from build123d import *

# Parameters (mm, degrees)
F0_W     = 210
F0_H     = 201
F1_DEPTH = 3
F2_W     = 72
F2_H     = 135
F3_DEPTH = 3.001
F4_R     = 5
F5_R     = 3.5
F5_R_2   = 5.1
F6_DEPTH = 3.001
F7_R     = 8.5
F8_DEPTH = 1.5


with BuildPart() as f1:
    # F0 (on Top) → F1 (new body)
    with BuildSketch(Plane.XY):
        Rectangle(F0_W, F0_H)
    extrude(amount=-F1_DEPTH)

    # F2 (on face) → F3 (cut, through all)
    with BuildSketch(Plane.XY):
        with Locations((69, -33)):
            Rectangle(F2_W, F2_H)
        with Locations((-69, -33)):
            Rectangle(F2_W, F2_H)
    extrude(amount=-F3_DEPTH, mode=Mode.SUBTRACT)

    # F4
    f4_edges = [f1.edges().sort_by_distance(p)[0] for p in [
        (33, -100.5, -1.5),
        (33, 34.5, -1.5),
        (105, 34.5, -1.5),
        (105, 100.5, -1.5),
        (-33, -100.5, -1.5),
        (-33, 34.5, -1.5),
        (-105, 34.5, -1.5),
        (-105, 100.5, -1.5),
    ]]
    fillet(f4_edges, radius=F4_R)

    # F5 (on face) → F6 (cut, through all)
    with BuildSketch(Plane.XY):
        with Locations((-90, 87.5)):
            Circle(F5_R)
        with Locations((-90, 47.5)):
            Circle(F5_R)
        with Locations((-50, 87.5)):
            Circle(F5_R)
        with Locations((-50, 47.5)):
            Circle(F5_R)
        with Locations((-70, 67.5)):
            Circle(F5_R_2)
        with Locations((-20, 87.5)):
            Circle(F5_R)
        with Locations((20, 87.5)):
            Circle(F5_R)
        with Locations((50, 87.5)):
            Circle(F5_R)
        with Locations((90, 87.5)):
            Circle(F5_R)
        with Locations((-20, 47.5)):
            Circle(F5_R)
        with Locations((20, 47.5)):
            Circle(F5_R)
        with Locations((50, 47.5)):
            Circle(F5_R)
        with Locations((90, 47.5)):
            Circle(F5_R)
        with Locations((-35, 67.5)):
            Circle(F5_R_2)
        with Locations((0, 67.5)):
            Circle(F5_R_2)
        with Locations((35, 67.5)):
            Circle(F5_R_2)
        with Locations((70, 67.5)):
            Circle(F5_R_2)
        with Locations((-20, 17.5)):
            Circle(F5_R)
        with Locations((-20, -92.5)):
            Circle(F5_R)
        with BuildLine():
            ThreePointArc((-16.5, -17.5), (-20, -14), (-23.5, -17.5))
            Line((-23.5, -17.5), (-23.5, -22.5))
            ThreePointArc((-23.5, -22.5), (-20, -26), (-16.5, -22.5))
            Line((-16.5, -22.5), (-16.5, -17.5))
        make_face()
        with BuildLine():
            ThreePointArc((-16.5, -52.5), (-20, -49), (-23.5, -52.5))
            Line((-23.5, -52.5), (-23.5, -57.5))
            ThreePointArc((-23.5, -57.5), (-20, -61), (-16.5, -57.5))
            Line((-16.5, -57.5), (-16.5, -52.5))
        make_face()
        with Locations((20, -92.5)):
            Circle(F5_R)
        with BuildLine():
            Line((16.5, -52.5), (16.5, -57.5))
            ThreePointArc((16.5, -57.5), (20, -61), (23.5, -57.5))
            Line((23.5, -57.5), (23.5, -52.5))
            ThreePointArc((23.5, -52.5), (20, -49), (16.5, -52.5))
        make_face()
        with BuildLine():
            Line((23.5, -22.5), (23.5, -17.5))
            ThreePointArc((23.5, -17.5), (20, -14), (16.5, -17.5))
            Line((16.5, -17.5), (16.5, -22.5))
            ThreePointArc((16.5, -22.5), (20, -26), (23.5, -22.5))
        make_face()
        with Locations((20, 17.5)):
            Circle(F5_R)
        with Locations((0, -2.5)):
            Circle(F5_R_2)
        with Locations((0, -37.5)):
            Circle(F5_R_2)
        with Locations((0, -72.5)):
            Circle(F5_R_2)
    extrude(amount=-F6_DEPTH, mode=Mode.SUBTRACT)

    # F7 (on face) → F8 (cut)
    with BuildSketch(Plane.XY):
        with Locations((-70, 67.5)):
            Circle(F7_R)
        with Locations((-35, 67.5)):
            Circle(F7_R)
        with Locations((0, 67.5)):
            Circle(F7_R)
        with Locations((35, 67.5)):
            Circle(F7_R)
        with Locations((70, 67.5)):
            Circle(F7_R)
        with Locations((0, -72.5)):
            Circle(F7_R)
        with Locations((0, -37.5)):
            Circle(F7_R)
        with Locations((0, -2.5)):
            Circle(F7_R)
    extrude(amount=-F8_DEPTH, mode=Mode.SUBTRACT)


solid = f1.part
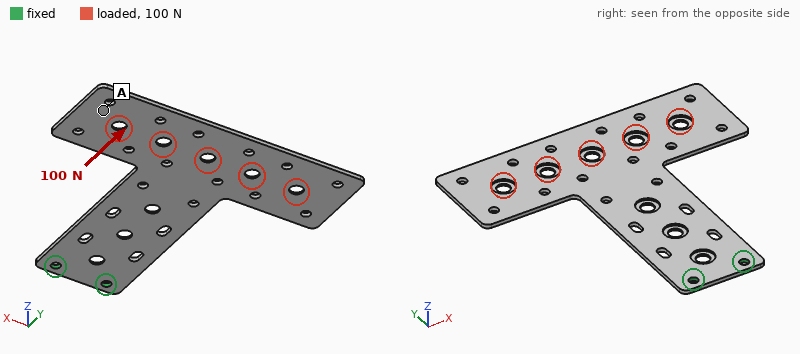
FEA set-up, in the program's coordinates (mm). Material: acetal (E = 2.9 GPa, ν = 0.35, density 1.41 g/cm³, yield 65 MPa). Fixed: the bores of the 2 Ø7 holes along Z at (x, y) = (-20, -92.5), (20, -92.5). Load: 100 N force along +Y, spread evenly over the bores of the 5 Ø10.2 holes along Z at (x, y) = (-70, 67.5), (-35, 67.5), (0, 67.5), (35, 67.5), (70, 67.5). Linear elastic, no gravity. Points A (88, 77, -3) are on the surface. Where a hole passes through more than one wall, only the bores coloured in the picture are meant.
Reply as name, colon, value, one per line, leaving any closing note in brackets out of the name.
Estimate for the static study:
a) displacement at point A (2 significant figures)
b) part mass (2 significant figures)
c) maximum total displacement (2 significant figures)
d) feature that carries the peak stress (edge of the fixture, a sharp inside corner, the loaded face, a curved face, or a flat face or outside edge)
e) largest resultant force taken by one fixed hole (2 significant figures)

displacement at point A: 2.7 mm
part mass: 87 g
maximum total displacement: 3.4 mm
feature that carries the peak stress: a curved face
largest resultant force taken by one fixed hole: 50 N
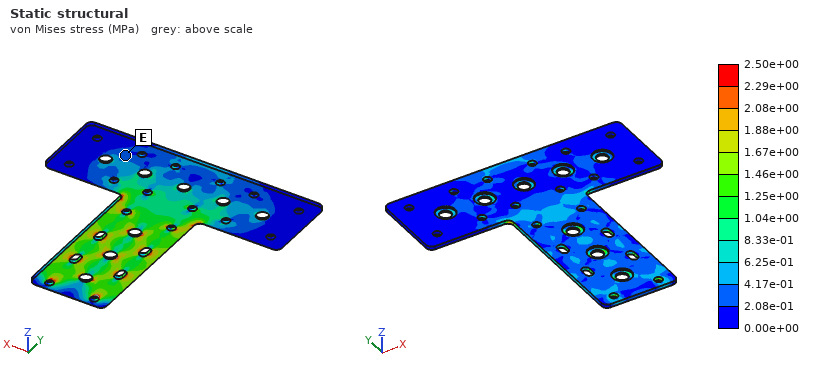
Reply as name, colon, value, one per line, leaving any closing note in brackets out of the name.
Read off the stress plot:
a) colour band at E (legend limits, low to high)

colour band at E: 2.08e-01 to 4.17e-01 MPa
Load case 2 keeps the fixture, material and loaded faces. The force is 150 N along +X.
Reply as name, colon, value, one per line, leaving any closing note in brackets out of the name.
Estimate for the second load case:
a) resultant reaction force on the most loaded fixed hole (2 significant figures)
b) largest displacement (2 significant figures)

resultant reaction force on the most loaded fixed hole: 540 N
largest displacement: 3.4 mm
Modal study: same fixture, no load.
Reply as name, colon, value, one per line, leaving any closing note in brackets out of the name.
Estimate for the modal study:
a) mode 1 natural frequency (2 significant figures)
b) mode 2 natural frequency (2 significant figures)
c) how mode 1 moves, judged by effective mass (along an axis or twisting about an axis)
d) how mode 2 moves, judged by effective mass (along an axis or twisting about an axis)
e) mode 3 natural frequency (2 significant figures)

mode 1 natural frequency: 11 Hz
mode 2 natural frequency: 23 Hz
how mode 1 moves, judged by effective mass: along Z
how mode 2 moves, judged by effective mass: twisting about Y
mode 3 natural frequency: 93 Hz
